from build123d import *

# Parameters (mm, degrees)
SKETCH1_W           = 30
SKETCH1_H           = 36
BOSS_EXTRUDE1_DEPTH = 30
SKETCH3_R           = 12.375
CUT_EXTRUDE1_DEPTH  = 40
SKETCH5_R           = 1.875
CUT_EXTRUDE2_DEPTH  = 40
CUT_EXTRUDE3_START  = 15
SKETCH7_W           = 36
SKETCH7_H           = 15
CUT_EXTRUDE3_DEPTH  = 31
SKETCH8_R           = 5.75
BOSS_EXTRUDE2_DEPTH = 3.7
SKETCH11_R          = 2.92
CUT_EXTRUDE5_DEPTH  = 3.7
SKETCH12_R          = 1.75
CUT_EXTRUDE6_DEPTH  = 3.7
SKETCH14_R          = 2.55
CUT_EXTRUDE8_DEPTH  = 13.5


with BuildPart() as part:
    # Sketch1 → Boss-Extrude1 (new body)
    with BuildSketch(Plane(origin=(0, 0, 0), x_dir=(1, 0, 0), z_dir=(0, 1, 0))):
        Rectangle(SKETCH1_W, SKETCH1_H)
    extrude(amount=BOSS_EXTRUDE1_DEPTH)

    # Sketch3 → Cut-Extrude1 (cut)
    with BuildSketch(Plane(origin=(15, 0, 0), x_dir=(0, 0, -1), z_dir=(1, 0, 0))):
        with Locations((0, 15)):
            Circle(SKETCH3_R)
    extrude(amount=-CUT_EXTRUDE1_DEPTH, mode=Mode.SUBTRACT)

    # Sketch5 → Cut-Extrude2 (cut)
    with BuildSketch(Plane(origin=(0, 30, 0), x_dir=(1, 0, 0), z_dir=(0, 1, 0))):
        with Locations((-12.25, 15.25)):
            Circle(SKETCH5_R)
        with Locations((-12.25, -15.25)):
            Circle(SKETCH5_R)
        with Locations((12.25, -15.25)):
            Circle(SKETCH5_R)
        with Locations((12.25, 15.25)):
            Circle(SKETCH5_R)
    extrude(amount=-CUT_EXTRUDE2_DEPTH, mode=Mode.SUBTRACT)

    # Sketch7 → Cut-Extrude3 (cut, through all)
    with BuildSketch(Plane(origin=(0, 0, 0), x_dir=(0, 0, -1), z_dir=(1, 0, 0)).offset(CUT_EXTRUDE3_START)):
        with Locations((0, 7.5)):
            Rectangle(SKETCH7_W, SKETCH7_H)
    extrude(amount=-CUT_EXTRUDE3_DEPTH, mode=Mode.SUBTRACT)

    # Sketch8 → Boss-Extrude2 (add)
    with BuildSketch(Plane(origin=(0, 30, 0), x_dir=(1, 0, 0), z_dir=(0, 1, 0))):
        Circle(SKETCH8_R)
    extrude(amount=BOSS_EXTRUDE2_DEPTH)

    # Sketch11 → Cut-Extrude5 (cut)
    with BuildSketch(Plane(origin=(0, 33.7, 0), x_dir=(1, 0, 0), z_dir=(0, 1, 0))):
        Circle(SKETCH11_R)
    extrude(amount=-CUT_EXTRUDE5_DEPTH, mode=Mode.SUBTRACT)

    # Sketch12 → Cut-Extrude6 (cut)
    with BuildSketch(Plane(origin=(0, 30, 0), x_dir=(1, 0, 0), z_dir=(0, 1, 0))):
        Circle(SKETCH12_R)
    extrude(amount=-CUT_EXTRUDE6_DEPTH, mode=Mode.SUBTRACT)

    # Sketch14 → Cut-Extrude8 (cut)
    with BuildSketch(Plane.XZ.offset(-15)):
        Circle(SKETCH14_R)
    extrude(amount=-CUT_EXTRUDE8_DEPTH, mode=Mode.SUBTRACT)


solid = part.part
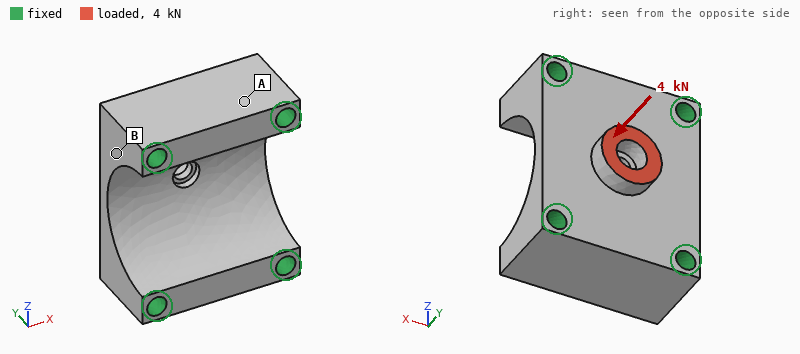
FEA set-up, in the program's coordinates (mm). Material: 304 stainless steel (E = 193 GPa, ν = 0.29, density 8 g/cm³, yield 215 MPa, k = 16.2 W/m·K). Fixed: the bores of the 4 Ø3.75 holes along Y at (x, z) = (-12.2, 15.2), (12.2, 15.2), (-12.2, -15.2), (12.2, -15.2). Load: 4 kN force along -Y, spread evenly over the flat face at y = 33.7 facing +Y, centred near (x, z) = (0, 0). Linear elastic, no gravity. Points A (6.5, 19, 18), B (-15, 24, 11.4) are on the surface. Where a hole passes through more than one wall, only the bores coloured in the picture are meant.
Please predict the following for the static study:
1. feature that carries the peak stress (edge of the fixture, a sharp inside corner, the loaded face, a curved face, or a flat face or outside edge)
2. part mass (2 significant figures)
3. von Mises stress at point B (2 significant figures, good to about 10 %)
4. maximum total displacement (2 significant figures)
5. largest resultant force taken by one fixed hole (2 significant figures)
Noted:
a curved face
69 g
19 MPa
9.0 µm
1.5 kN
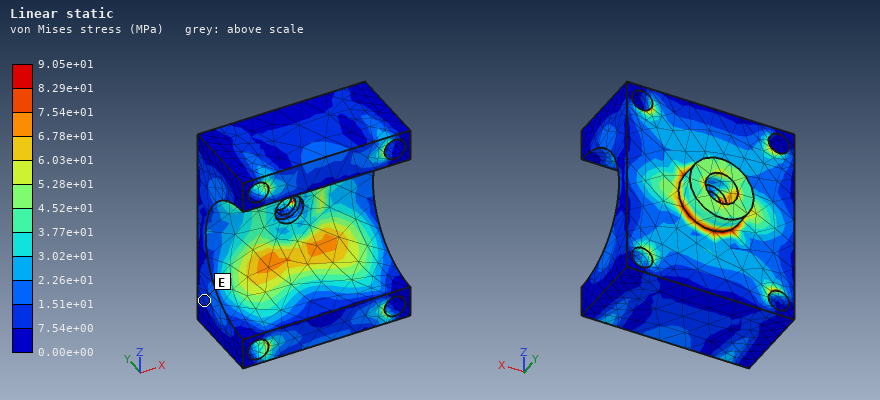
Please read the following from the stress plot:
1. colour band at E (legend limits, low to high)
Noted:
7.54e+00 to 1.51e+01 MPa
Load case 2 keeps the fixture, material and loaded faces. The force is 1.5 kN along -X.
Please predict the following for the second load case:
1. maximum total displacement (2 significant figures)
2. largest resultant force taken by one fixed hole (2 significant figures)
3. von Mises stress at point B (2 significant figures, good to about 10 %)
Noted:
6.4 µm
630 N
12 MPa
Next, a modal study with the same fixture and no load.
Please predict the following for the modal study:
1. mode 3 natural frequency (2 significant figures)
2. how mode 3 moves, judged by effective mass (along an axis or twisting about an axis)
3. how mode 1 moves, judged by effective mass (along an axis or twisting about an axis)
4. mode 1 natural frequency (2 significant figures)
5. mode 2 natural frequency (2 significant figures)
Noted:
47 kHz
along Z
along Y
36 kHz
45 kHz
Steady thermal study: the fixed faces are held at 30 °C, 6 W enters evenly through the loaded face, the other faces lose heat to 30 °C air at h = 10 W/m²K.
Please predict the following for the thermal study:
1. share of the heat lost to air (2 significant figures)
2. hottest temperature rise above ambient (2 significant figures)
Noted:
4.1 %
42 K
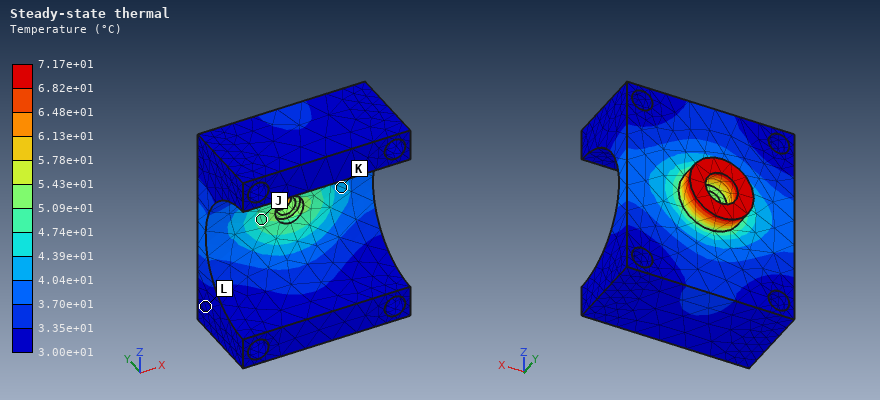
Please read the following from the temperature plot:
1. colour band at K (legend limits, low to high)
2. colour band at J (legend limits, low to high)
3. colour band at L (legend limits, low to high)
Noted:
4.04e+01 to 4.39e+01 °C
4.74e+01 to 5.09e+01 °C
3.00e+01 to 3.35e+01 °C
